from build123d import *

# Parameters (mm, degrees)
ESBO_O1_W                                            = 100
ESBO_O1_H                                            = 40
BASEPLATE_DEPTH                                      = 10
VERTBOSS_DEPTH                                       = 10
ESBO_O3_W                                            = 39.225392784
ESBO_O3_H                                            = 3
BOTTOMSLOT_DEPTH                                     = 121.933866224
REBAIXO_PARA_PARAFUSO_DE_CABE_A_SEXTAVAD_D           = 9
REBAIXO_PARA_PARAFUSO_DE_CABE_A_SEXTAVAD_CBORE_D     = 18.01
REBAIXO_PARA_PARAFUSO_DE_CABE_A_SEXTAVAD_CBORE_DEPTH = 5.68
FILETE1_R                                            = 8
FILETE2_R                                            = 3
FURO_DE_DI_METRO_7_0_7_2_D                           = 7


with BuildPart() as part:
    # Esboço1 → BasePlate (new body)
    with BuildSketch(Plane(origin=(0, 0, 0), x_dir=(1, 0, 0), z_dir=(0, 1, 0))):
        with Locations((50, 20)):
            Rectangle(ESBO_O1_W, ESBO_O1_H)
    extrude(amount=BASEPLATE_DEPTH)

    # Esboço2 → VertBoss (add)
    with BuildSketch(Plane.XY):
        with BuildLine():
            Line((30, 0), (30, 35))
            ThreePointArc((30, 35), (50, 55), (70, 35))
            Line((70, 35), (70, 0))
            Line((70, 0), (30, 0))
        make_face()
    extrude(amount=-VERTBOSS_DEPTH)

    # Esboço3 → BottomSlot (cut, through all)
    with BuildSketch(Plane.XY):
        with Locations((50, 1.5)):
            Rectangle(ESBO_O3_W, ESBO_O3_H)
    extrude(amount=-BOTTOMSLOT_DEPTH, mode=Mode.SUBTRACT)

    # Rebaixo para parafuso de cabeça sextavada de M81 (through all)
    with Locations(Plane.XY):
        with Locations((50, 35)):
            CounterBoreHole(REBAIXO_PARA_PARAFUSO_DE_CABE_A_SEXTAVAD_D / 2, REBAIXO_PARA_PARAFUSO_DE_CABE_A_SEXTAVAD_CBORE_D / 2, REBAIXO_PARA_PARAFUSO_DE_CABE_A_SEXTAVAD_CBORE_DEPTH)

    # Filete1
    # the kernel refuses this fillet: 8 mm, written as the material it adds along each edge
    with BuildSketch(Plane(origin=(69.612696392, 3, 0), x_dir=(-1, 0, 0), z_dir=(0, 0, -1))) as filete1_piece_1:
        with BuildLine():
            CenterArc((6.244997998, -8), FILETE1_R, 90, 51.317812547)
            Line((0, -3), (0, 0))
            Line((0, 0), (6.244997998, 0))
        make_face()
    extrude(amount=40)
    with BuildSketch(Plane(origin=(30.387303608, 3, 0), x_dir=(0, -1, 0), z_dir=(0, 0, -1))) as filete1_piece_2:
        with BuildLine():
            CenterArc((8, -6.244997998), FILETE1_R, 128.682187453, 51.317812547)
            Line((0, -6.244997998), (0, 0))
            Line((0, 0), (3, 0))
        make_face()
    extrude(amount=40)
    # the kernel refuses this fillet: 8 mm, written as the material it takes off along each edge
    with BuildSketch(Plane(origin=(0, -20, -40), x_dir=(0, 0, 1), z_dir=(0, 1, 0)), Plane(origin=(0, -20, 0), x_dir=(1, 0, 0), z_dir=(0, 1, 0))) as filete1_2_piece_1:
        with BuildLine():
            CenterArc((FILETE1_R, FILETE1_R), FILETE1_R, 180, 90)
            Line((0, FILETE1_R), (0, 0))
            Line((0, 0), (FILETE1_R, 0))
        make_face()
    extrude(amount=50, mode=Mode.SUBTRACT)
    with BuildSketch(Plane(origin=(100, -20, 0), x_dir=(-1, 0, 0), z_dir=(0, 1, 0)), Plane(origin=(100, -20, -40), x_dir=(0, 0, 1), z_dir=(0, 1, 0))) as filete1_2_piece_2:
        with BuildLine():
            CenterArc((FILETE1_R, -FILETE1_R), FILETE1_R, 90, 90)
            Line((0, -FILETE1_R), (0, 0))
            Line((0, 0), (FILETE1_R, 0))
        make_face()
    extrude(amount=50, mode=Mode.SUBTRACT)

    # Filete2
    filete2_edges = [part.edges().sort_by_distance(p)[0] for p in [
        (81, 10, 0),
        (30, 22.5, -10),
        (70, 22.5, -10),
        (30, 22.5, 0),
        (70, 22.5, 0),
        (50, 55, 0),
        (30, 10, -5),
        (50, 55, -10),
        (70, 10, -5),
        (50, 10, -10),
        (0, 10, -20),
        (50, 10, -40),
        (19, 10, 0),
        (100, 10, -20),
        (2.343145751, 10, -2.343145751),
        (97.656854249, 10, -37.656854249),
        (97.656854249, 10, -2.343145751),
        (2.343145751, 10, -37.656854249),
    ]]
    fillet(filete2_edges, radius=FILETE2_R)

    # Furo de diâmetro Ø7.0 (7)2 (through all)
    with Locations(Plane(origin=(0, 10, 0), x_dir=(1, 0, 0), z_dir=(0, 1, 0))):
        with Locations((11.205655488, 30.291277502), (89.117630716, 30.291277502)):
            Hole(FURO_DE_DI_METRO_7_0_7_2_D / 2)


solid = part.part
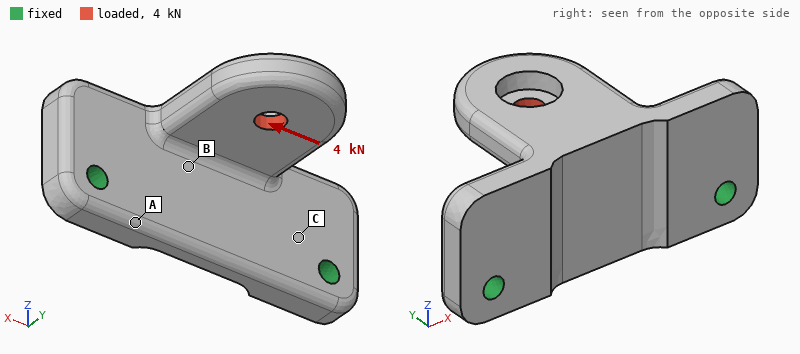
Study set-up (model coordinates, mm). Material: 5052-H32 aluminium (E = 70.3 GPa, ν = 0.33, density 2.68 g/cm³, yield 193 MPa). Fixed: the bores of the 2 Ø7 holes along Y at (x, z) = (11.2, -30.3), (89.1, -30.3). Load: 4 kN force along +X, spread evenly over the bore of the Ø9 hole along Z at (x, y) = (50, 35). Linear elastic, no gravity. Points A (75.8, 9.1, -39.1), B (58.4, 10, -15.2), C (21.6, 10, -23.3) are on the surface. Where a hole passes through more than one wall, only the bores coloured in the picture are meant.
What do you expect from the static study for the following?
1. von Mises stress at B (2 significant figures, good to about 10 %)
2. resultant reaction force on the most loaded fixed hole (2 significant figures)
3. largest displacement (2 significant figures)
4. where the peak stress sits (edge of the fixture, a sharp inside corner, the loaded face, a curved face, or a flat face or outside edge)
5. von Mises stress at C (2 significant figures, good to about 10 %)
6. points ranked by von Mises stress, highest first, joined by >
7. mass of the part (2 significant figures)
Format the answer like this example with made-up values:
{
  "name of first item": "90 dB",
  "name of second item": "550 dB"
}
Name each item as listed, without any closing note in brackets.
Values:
{
  "von Mises stress at B": "54 MPa",
  "resultant reaction force on the most loaded fixed hole": "3.0 kN",
  "largest displacement": "0.17 mm",
  "where the peak stress sits": "a curved face",
  "von Mises stress at C": "30 MPa",
  "points ranked by von Mises stress, highest first, joined by >": "B > C > A",
  "mass of the part": "130 g"
}
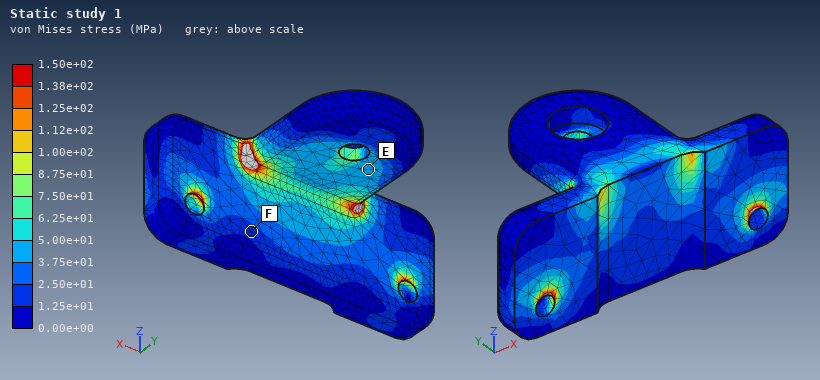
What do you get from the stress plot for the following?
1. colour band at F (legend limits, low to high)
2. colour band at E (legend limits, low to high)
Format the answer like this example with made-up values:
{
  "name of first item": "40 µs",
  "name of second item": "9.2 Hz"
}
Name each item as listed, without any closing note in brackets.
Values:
{
  "colour band at F": "1.25e+01 to 2.50e+01 MPa",
  "colour band at E": "3.75e+01 to 5.00e+01 MPa"
}
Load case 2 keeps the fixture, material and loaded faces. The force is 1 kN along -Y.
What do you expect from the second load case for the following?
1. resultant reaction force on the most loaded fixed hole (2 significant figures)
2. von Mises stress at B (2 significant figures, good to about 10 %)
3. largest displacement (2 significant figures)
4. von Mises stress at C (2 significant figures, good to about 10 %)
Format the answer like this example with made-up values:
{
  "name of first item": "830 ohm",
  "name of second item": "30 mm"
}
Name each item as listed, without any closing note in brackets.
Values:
{
  "resultant reaction force on the most loaded fixed hole": "530 N",
  "von Mises stress at B": "3.9 MPa",
  "largest displacement": "48 µm",
  "von Mises stress at C": "13 MPa"
}
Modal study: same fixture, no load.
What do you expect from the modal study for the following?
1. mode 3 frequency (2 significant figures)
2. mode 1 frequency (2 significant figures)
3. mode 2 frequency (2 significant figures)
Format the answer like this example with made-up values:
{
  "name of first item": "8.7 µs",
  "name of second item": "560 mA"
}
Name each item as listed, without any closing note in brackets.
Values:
{
  "mode 3 frequency": "4800 Hz",
  "mode 1 frequency": "2300 Hz",
  "mode 2 frequency": "4800 Hz"
}
